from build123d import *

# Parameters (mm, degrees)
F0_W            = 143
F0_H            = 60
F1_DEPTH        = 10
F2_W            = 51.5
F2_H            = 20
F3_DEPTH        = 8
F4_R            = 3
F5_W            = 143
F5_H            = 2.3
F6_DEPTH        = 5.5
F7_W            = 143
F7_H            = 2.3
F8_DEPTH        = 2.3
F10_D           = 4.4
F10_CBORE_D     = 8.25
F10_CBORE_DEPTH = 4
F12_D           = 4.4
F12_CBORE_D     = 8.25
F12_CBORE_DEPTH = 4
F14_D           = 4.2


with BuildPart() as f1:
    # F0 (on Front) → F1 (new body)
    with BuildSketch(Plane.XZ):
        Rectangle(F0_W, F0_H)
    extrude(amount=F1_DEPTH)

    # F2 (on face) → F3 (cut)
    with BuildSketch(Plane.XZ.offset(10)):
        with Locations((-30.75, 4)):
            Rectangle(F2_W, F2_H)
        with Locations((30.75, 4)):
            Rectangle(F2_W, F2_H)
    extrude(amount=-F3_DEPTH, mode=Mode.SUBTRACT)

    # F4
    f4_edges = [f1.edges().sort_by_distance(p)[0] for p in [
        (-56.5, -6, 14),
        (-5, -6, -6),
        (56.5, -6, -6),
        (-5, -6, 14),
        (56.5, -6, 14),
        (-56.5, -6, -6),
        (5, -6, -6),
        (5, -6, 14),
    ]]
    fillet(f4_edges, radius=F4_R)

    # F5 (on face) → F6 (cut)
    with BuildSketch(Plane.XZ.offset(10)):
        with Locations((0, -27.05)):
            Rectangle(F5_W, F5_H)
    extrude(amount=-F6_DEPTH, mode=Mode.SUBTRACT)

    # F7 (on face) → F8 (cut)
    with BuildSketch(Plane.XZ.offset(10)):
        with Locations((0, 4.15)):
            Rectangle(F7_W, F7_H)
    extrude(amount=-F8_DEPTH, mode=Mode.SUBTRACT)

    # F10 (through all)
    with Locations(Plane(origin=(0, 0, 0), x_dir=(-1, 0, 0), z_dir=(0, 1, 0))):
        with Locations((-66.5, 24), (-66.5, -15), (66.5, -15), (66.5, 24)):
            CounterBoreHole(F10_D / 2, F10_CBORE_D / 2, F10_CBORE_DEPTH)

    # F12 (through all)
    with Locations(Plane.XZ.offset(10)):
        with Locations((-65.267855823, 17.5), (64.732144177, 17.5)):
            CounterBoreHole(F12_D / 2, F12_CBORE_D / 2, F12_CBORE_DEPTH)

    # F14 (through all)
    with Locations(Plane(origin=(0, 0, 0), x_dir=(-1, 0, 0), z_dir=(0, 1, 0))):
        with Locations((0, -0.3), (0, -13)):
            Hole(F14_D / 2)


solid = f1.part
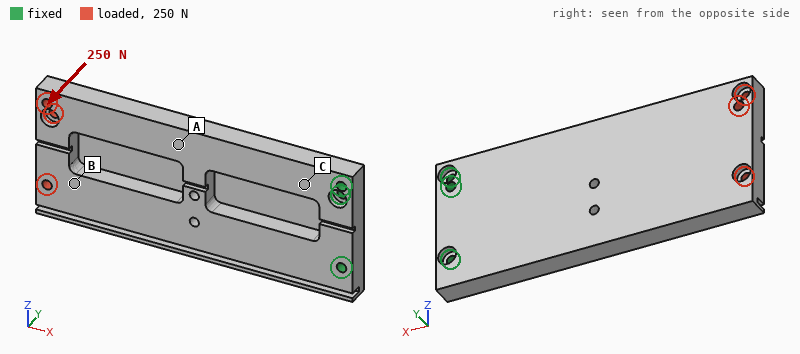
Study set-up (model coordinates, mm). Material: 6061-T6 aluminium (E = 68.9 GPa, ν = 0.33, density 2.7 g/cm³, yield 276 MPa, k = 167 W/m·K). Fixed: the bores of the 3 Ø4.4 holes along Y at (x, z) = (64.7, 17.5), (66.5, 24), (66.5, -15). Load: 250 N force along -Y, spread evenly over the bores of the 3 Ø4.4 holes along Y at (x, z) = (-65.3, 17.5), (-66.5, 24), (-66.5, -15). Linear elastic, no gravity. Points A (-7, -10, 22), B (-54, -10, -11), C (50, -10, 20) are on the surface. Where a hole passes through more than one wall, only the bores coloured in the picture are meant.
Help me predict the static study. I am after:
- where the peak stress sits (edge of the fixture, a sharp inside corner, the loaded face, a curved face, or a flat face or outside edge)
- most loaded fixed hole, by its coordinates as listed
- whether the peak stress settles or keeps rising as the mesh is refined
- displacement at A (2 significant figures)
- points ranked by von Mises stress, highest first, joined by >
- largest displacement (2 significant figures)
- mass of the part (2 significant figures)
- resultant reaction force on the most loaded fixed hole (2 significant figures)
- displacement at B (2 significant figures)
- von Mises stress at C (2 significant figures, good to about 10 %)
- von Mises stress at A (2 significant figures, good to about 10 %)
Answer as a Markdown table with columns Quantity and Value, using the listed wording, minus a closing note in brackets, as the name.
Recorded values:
| Quantity | Value |
|---|---|
| where the peak stress sits | edge of the fixture |
| most loaded fixed hole, by its coordinates as listed | (64.7, 17.5) |
| whether the peak stress settles or keeps rising as the mesh is refined | keeps rising |
| displacement at A | 0.35 mm |
| points ranked by von Mises stress, highest first, joined by > | C > A > B |
| largest displacement | 0.94 mm |
| mass of the part | 180 g |
| resultant reaction force on the most loaded fixed hole | 1.9 kN |
| displacement at B | 0.75 mm |
| von Mises stress at C | 45 MPa |
| von Mises stress at A | 21 MPa |
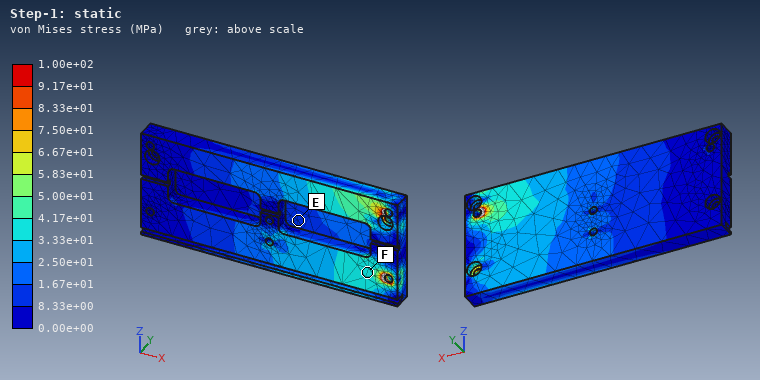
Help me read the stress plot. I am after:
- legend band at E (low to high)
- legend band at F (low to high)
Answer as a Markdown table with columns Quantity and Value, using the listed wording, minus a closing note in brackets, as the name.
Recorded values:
| Quantity | Value |
|---|---|
| legend band at E | 8.33e+00 to 1.67e+01 MPa |
| legend band at F | 3.33e+01 to 4.17e+01 MPa |
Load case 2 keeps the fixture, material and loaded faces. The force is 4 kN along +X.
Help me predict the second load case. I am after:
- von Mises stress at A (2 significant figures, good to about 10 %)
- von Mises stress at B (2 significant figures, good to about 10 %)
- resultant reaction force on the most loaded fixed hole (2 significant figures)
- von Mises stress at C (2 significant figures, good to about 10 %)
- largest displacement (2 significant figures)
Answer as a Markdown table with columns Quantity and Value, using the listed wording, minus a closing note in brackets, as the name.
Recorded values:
| Quantity | Value |
|---|---|
| von Mises stress at A | 21 MPa |
| von Mises stress at B | 14 MPa |
| resultant reaction force on the most loaded fixed hole | 1.4 kN |
| von Mises stress at C | 20 MPa |
| largest displacement | 0.16 mm |
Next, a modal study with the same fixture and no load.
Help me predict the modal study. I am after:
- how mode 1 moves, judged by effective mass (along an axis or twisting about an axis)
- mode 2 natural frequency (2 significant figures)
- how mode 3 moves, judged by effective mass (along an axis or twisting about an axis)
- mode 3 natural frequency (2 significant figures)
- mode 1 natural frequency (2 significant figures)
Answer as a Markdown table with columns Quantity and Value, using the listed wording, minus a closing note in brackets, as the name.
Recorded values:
| Quantity | Value |
|---|---|
| how mode 1 moves, judged by effective mass | along Y |
| mode 2 natural frequency | 1400 Hz |
| how mode 3 moves, judged by effective mass | along Z |
| mode 3 natural frequency | 2000 Hz |
| mode 1 natural frequency | 380 Hz |
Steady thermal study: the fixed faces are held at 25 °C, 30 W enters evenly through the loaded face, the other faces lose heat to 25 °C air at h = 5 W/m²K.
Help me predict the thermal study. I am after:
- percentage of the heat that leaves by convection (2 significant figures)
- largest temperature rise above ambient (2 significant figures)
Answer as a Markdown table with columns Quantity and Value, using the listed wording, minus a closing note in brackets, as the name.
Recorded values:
| Quantity | Value |
|---|---|
| percentage of the heat that leaves by convection | 11 % |
| largest temperature rise above ambient | 60 K |
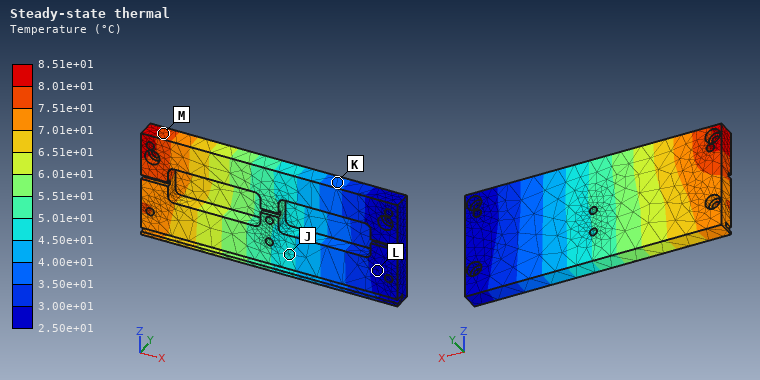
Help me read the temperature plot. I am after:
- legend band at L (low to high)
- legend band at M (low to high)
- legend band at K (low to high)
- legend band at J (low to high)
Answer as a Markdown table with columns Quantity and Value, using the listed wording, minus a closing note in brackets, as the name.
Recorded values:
| Quantity | Value |
|---|---|
| legend band at L | 2.50e+01 to 3.00e+01 °C |
| legend band at M | 7.51e+01 to 8.01e+01 °C |
| legend band at K | 3.50e+01 to 4.00e+01 °C |
| legend band at J | 4.50e+01 to 5.01e+01 °C |
